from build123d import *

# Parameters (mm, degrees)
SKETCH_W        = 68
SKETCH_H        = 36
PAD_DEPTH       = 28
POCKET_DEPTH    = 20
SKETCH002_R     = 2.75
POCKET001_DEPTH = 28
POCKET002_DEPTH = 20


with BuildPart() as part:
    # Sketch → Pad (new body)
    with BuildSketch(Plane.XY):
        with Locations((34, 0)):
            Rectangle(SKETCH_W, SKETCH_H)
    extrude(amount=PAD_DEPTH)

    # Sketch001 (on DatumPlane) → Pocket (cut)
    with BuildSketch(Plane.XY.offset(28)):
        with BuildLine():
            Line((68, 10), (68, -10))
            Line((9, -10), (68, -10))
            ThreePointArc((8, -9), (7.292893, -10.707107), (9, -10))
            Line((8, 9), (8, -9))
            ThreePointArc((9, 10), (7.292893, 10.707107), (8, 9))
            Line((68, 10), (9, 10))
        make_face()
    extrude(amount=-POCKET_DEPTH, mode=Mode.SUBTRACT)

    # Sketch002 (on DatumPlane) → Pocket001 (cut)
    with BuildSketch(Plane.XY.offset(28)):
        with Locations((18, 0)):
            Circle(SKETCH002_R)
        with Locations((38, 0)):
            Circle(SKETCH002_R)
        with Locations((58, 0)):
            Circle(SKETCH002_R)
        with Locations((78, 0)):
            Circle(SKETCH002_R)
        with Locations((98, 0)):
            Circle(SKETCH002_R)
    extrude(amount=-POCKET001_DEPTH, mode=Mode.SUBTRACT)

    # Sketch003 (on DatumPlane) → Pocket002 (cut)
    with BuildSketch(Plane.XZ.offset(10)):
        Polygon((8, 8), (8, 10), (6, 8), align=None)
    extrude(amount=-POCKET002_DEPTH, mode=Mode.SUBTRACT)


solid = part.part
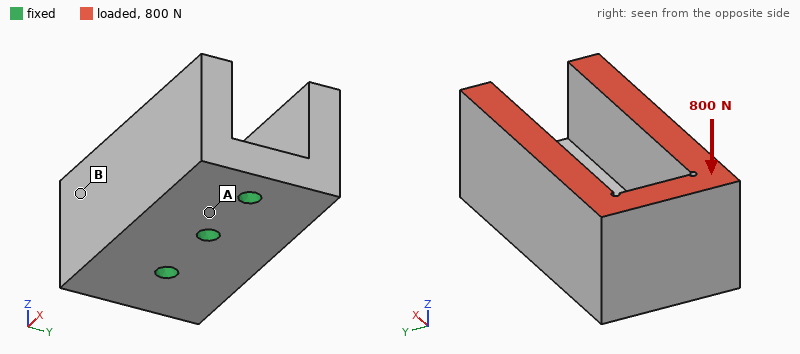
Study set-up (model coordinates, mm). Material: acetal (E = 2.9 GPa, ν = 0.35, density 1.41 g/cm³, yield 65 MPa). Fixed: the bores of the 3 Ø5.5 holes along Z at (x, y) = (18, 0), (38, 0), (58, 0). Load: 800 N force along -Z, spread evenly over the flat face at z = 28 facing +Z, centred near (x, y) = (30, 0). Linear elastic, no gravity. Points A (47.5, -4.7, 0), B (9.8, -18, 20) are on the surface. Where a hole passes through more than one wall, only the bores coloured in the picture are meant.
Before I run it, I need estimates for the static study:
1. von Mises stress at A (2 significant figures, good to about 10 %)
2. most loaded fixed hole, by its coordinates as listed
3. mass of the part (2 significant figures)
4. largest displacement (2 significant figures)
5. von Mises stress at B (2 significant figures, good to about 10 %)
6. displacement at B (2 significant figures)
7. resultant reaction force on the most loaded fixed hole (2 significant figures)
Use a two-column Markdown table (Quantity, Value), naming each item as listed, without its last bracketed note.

| Quantity | Value |
|---|---|
| von Mises stress at A | 2.7 MPa |
| most loaded fixed hole, by its coordinates as listed | (18, 0) |
| mass of the part | 62 g |
| largest displacement | 79 µm |
| von Mises stress at B | 0.82 MPa |
| displacement at B | 45 µm |
| resultant reaction force on the most loaded fixed hole | 430 N |
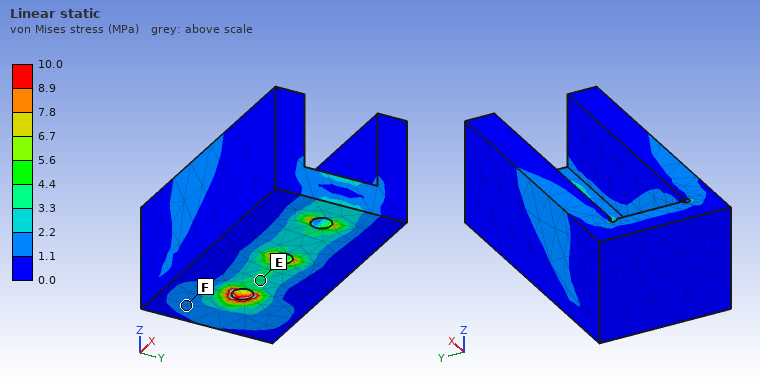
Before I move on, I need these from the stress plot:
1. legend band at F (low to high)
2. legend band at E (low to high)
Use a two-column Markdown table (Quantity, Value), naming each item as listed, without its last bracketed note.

| Quantity | Value |
|---|---|
| legend band at F | 1.1 to 2.2 MPa |
| legend band at E | 3.3 to 4.4 MPa |
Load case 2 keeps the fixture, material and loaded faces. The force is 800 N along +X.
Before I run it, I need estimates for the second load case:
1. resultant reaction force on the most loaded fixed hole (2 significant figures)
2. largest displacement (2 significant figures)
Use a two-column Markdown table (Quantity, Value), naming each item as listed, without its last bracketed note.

| Quantity | Value |
|---|---|
| resultant reaction force on the most loaded fixed hole | 510 N |
| largest displacement | 0.14 mm |
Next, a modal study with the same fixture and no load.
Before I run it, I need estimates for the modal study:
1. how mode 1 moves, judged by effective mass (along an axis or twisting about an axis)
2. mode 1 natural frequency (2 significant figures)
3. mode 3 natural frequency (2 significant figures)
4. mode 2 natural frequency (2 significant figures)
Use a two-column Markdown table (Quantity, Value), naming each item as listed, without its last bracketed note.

| Quantity | Value |
|---|---|
| how mode 1 moves, judged by effective mass | along Y |
| mode 1 natural frequency | 1500 Hz |
| mode 3 natural frequency | 2300 Hz |
| mode 2 natural frequency | 2100 Hz |
